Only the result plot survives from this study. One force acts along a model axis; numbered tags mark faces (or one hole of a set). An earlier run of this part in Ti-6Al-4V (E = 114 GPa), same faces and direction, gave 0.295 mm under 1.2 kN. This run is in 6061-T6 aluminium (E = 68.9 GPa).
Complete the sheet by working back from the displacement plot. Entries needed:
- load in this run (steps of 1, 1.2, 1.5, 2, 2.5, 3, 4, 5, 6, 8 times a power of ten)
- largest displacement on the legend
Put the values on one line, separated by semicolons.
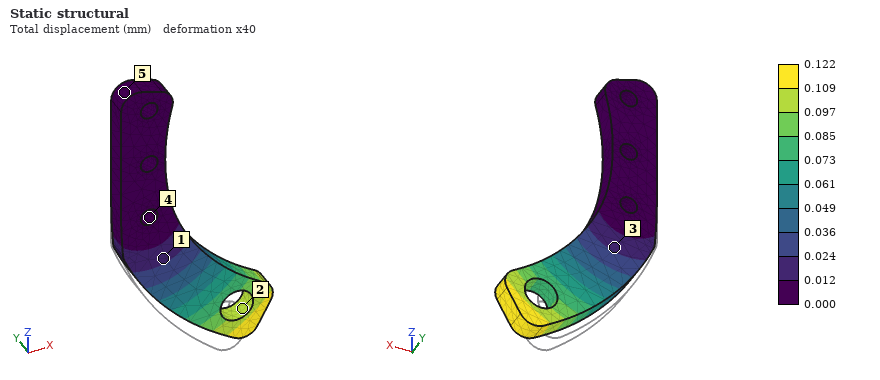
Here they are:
300 N; 0.122 mm
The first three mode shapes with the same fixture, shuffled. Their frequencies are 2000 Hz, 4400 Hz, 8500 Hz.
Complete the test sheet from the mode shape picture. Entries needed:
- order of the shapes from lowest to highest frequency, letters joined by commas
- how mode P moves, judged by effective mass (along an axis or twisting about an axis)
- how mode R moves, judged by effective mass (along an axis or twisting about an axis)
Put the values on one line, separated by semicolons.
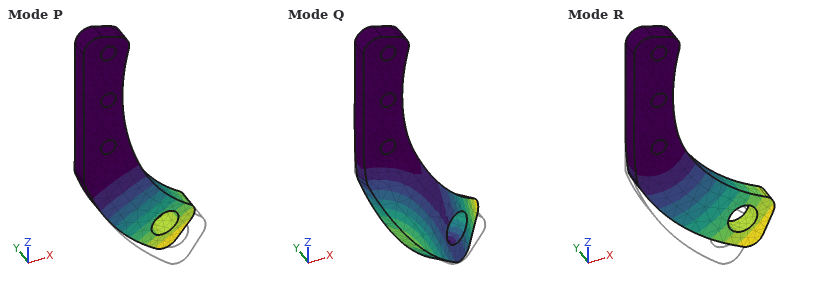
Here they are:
P, R, Q; along Y; along X
